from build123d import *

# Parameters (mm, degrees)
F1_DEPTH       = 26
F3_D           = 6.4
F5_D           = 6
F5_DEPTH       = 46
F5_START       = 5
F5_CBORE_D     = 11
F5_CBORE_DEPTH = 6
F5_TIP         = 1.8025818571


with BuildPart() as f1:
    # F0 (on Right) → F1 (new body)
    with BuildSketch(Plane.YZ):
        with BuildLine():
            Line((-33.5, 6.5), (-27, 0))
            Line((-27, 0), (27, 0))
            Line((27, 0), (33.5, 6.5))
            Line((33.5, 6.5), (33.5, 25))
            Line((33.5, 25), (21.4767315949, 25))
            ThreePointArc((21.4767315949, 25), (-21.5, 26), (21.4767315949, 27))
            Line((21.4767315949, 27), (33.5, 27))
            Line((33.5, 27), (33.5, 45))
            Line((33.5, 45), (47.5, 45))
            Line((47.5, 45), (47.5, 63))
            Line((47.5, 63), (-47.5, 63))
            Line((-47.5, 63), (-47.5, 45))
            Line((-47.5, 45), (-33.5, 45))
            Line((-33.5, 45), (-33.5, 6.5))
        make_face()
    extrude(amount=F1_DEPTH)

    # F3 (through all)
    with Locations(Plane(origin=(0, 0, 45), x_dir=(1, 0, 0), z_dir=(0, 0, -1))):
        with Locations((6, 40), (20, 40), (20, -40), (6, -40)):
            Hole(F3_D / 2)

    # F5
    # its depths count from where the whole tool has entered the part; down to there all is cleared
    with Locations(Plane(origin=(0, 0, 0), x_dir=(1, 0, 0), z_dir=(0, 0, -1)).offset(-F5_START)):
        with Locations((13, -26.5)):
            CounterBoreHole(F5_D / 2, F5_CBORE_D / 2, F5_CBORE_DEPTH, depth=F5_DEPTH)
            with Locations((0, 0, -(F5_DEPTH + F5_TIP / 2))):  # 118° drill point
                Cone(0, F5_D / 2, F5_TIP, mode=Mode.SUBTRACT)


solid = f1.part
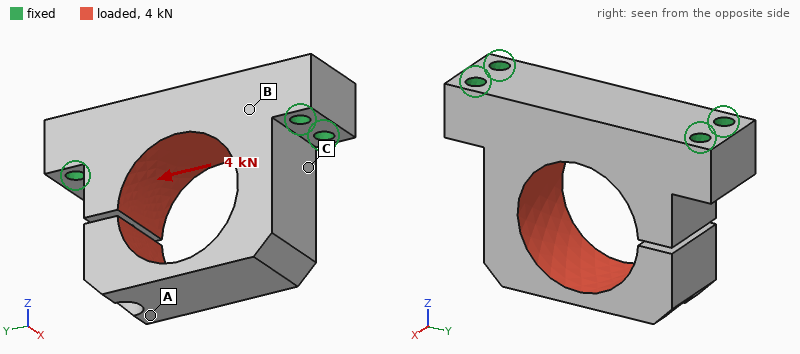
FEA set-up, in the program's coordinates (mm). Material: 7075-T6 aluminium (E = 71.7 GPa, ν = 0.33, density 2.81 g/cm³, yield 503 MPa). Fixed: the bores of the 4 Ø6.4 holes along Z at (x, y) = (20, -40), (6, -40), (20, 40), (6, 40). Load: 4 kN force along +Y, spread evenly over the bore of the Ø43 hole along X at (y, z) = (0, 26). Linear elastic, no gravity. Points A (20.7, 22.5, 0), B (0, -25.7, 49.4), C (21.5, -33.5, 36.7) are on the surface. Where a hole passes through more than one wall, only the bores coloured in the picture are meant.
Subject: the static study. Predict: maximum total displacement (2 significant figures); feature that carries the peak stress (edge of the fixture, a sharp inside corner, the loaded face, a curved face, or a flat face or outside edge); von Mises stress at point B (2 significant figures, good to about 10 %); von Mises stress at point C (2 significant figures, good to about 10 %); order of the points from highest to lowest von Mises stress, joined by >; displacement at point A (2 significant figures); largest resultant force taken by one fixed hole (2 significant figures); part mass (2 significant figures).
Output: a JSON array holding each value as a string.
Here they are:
["0.30 mm", "the loaded face", "24 MPa", "53 MPa", "C > B > A", "0.12 mm", "1.6 kN", "220 g"]
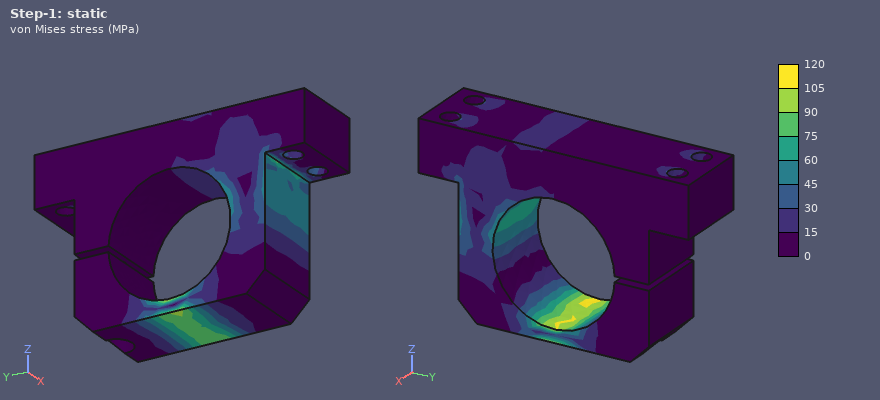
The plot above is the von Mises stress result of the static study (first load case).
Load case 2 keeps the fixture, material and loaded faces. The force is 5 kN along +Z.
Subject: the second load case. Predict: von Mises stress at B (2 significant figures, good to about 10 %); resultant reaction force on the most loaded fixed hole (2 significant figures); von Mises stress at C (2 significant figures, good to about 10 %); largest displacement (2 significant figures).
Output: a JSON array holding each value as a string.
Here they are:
["36 MPa", "1.4 kN", "67 MPa", "1.3 mm"]
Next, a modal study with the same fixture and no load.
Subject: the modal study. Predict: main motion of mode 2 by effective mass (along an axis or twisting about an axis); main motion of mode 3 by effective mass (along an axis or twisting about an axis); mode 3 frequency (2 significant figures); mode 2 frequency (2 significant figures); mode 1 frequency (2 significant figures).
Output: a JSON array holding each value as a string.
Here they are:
["along X", "along Y", "2200 Hz", "1500 Hz", "920 Hz"]
